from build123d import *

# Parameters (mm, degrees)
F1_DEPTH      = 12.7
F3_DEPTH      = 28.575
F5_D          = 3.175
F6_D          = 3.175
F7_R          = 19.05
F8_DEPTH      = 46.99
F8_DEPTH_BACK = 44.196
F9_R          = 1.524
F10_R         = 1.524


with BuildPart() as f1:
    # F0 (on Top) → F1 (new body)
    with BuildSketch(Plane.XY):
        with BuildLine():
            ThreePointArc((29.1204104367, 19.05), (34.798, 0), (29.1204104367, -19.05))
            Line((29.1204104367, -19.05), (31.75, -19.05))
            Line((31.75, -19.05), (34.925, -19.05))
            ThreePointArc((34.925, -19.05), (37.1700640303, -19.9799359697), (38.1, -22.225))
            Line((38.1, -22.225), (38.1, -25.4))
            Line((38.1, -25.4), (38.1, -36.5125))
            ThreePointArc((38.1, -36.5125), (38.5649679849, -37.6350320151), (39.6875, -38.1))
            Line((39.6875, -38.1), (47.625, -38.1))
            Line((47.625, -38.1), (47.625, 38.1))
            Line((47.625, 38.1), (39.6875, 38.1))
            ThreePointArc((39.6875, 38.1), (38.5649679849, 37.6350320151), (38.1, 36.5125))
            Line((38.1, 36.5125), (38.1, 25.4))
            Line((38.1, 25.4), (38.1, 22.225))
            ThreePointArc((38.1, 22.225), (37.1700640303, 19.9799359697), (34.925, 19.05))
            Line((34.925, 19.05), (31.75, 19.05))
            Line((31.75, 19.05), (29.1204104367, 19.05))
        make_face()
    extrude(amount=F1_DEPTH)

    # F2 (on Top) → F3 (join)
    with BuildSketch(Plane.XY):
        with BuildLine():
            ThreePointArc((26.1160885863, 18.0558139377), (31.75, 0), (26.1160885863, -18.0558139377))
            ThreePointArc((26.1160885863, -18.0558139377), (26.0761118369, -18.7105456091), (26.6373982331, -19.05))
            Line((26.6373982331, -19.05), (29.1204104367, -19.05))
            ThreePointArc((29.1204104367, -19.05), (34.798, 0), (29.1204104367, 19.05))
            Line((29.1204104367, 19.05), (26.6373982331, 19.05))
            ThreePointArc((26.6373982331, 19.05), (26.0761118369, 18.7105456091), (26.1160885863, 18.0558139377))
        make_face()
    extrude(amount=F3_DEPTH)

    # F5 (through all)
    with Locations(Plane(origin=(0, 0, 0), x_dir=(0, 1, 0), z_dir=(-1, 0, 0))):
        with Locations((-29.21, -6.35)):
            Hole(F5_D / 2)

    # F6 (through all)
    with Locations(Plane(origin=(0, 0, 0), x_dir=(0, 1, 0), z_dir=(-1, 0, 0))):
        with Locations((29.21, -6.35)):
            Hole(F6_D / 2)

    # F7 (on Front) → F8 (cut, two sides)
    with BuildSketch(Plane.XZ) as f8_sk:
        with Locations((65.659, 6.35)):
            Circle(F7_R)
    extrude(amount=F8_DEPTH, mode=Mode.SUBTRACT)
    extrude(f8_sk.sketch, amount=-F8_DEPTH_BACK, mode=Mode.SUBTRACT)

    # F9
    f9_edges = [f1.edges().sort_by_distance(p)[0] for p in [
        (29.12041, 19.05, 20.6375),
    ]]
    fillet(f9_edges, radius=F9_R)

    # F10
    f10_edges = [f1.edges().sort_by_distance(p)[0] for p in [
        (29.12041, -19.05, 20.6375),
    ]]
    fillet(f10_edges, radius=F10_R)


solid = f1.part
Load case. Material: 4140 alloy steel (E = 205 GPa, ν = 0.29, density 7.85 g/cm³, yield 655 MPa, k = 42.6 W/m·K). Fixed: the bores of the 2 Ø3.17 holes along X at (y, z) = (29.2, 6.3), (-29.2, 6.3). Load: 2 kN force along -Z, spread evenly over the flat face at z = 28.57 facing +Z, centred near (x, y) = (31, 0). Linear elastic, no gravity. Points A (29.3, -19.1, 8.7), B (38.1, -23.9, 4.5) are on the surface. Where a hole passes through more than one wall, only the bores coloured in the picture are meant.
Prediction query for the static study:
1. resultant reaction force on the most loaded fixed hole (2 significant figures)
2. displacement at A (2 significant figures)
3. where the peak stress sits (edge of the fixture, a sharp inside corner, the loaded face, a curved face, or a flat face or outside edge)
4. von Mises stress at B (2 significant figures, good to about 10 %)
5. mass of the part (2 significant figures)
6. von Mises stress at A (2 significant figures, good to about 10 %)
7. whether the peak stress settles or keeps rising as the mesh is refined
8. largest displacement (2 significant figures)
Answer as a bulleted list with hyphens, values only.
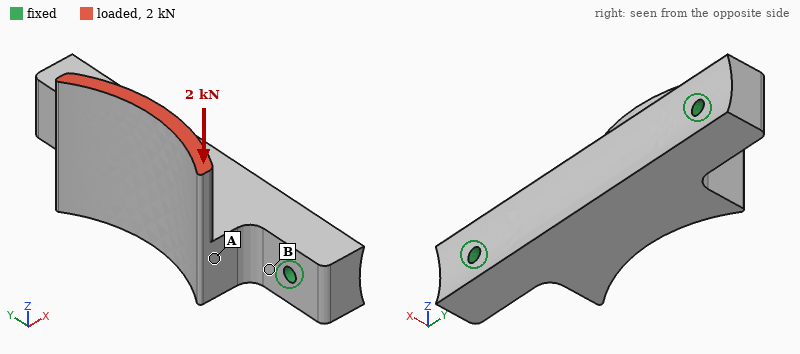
- 1.0 kN
- 20 µm
- edge of the fixture
- 96 MPa
- 110 g
- 21 MPa
- keeps rising
- 35 µm
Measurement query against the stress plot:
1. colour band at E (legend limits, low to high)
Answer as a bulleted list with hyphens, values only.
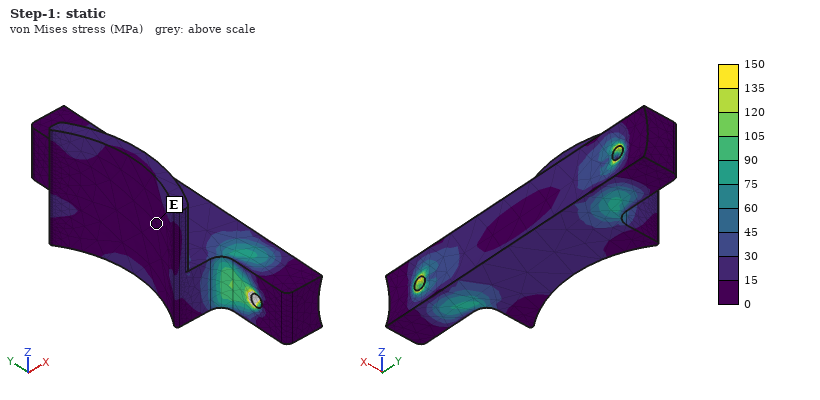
- 0 to 15 MPa
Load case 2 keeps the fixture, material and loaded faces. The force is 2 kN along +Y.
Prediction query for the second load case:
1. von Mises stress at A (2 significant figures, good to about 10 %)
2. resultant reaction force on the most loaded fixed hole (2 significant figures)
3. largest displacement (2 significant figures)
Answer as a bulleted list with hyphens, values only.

- 31 MPa
- 1.4 kN
- 39 µm
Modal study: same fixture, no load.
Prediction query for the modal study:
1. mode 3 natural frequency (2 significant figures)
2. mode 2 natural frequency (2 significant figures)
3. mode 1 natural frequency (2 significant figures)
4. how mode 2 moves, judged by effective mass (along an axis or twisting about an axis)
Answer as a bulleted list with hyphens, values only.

- 11 kHz
- 9100 Hz
- 6400 Hz
- along Z
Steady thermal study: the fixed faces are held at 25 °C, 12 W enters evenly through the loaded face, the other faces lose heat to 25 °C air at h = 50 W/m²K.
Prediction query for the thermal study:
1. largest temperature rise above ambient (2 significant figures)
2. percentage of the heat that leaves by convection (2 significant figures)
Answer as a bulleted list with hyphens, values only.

- 52 K
- 36 %
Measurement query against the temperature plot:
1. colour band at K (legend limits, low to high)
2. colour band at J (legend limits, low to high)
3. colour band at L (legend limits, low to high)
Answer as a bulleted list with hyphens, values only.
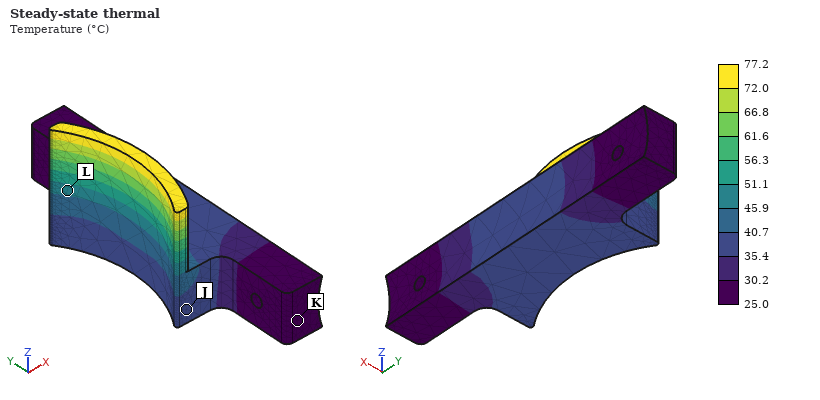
- 25.0 to 30.2 °C
- 35.4 to 40.7 °C
- 45.9 to 51.1 °C
